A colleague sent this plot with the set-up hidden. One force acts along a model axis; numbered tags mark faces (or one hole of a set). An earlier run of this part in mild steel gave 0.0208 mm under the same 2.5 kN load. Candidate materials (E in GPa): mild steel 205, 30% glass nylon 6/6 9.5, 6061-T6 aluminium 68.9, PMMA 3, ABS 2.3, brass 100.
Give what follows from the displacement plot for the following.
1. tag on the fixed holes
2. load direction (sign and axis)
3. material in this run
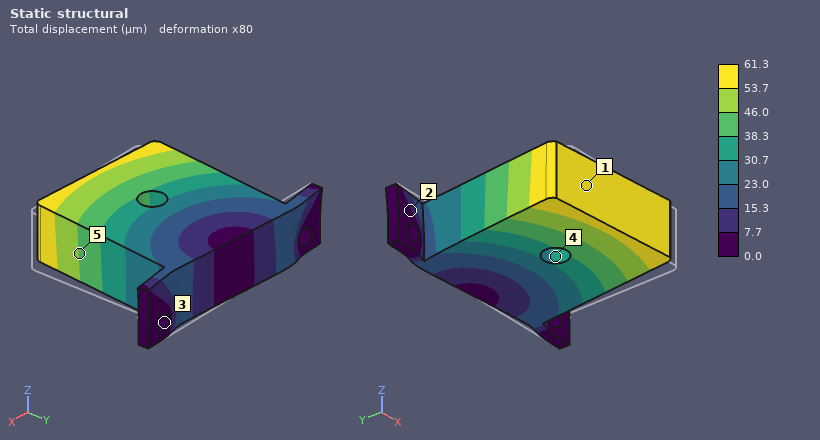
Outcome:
3
-X
6061-T6 aluminium
